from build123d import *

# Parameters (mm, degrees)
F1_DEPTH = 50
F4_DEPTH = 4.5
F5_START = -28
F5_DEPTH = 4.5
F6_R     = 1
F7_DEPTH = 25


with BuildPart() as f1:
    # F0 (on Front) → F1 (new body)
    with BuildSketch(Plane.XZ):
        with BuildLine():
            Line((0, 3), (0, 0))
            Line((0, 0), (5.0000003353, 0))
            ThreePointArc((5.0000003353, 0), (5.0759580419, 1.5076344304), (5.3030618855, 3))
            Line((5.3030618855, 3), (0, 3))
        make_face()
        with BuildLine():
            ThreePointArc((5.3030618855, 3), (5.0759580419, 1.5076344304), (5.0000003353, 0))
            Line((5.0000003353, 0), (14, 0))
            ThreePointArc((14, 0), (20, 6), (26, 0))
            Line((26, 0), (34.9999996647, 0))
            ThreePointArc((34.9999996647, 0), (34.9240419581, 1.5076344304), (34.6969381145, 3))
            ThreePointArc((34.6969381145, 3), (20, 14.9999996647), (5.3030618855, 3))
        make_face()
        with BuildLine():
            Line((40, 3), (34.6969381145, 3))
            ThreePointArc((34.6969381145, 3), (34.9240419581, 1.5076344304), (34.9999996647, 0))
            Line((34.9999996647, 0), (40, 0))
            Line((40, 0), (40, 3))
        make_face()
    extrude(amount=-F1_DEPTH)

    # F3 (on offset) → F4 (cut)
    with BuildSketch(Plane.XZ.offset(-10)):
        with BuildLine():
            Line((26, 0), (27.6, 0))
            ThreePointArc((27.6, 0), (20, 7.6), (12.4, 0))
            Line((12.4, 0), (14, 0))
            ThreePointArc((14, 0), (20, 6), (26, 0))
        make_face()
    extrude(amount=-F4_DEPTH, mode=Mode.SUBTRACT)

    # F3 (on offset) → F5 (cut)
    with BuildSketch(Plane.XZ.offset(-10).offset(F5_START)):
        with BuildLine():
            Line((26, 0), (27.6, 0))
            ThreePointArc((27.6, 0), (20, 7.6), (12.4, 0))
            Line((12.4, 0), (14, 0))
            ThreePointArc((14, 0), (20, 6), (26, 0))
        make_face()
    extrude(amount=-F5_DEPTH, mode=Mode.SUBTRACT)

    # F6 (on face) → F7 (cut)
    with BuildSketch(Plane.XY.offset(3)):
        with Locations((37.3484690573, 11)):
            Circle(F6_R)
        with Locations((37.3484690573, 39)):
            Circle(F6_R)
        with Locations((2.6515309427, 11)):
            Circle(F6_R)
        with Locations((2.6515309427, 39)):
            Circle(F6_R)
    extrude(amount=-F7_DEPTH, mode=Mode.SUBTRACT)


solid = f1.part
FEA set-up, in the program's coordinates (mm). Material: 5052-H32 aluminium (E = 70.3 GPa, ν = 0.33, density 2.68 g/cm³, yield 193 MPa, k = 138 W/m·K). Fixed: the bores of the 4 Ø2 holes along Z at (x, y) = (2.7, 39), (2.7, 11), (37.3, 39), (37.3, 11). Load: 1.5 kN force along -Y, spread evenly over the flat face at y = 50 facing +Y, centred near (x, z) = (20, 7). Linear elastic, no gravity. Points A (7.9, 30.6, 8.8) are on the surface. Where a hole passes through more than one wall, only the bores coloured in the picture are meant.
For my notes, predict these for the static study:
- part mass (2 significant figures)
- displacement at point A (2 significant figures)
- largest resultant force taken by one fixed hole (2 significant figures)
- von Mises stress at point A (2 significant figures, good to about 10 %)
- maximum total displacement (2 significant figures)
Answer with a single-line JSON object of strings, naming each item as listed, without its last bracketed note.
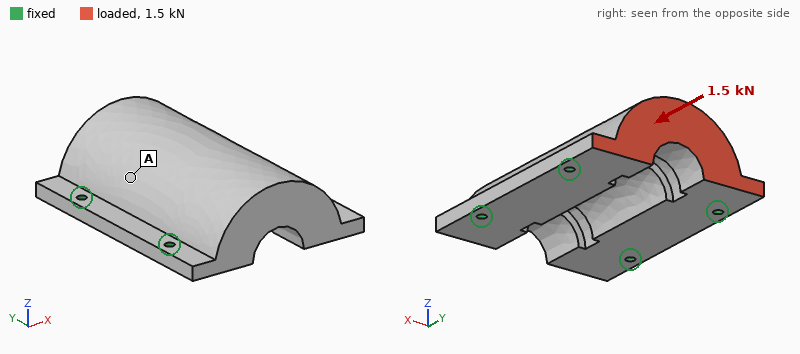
{"part mass": "43 g", "displacement at point A": "3.2 µm", "largest resultant force taken by one fixed hole": "480 N", "von Mises stress at point A": "5.3 MPa", "maximum total displacement": "7.9 µm"}
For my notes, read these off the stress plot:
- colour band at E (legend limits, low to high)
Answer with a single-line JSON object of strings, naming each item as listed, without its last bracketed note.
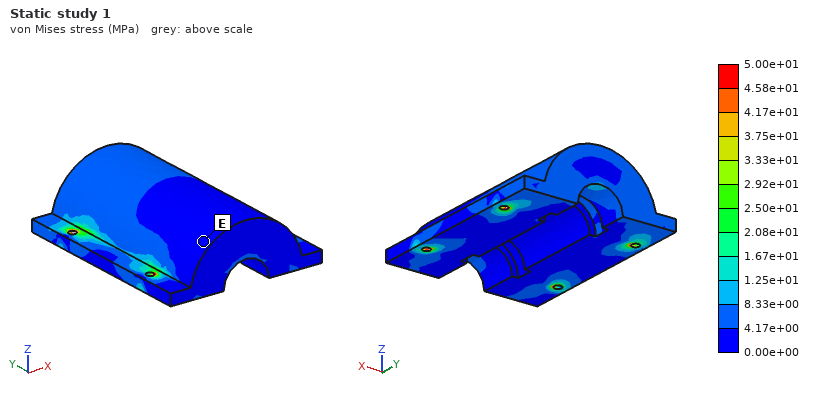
{"colour band at E": "0.00e+00 to 4.17e+00 MPa"}
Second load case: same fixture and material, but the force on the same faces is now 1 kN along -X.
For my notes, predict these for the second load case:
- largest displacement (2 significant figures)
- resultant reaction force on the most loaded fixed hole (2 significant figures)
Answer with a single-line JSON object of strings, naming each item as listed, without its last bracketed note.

{"largest displacement": "6.2 µm", "resultant reaction force on the most loaded fixed hole": "550 N"}
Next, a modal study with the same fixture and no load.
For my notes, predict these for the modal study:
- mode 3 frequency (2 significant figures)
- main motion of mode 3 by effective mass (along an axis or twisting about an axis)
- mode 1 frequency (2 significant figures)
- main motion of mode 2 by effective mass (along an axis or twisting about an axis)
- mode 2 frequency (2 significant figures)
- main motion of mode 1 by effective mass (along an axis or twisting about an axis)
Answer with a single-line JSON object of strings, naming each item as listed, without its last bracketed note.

{"mode 3 frequency": "20 kHz", "main motion of mode 3 by effective mass": "along X", "mode 1 frequency": "11 kHz", "main motion of mode 2 by effective mass": "along Z", "mode 2 frequency": "13 kHz", "main motion of mode 1 by effective mass": "along Y"}
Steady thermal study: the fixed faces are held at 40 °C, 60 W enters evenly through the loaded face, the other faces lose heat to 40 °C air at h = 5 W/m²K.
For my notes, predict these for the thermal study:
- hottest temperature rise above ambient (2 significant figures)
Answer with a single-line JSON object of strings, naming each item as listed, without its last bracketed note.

{"hottest temperature rise above ambient": "38 K"}
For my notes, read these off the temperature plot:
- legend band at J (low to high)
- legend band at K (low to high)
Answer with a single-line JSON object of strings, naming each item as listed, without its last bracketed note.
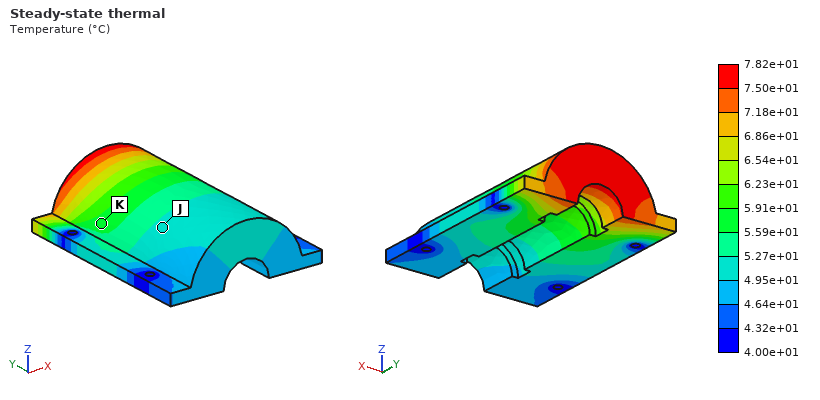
{"legend band at J": "4.95e+01 to 5.27e+01 °C", "legend band at K": "5.59e+01 to 5.91e+01 °C"}
